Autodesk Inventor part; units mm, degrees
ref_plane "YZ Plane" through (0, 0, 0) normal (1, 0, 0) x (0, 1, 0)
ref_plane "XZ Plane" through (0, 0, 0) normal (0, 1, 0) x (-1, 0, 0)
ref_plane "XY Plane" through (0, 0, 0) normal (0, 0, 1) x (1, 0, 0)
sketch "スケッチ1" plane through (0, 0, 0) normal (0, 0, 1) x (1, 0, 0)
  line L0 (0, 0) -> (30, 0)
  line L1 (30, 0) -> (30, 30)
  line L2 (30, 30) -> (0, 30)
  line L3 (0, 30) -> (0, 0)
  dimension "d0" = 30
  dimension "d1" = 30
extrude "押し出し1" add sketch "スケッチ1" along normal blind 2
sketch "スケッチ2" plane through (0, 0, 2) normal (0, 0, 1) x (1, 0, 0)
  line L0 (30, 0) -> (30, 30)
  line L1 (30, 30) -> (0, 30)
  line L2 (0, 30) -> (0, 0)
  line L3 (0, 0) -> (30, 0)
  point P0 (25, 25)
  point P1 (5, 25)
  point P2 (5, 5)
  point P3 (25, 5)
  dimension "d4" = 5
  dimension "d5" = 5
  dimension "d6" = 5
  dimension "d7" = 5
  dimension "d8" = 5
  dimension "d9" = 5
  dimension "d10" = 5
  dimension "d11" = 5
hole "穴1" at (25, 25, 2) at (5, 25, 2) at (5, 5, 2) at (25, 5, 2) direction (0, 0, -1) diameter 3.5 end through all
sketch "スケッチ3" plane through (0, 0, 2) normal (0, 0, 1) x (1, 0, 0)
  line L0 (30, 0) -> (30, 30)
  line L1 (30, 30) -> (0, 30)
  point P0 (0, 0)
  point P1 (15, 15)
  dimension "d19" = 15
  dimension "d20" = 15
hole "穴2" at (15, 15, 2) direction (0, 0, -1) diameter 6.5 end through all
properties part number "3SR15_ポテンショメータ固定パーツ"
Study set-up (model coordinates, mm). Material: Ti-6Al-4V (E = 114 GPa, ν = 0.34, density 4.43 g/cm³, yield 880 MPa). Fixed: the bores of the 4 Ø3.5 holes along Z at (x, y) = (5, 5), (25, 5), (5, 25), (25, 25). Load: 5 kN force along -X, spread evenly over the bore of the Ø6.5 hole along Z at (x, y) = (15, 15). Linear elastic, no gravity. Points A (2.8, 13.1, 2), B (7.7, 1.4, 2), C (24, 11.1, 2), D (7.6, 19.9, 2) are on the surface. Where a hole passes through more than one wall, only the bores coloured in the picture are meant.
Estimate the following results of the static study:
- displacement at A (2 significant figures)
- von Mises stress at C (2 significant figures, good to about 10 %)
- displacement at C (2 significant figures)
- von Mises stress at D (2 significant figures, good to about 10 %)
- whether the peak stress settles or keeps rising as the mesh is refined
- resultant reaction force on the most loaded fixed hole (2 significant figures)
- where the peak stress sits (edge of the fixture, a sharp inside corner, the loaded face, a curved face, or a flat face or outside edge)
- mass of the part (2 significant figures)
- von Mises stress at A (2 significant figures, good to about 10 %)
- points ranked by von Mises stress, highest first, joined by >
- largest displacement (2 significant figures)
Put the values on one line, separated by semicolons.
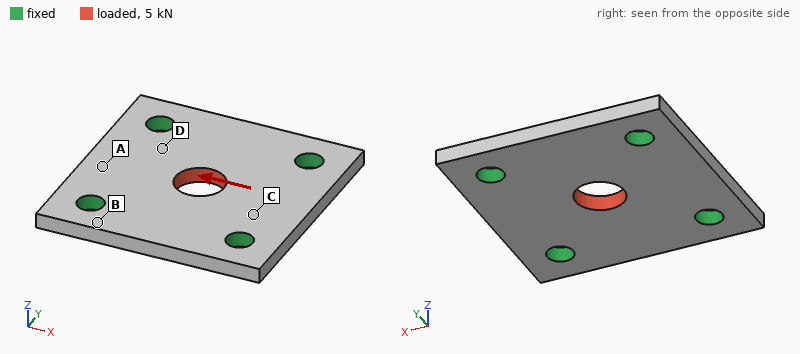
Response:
6.9 µm; 66 MPa; 6.1 µm; 90 MPa; keeps rising; 1.4 kN; edge of the fixture; 7.3 g; 32 MPa; D > C > A > B; 12 µm
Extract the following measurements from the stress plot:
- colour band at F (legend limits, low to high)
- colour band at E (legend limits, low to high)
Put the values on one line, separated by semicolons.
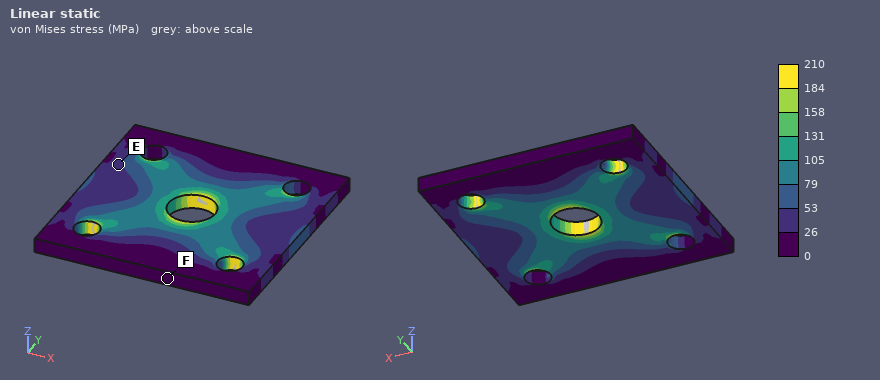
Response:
0 to 26 MPa; 26 to 53 MPa
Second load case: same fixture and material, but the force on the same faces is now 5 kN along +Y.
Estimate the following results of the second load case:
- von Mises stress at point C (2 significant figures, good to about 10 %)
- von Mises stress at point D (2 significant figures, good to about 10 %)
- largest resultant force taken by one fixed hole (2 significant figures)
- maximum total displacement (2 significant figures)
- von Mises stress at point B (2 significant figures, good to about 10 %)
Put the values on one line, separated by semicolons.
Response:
53 MPa; 83 MPa; 1.4 kN; 12 µm; 37 MPa
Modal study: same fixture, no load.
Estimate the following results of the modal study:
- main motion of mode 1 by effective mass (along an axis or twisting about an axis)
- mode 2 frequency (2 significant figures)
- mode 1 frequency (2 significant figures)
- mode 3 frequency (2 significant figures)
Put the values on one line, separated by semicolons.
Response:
along Z; 30 kHz; 23 kHz; 30 kHz
